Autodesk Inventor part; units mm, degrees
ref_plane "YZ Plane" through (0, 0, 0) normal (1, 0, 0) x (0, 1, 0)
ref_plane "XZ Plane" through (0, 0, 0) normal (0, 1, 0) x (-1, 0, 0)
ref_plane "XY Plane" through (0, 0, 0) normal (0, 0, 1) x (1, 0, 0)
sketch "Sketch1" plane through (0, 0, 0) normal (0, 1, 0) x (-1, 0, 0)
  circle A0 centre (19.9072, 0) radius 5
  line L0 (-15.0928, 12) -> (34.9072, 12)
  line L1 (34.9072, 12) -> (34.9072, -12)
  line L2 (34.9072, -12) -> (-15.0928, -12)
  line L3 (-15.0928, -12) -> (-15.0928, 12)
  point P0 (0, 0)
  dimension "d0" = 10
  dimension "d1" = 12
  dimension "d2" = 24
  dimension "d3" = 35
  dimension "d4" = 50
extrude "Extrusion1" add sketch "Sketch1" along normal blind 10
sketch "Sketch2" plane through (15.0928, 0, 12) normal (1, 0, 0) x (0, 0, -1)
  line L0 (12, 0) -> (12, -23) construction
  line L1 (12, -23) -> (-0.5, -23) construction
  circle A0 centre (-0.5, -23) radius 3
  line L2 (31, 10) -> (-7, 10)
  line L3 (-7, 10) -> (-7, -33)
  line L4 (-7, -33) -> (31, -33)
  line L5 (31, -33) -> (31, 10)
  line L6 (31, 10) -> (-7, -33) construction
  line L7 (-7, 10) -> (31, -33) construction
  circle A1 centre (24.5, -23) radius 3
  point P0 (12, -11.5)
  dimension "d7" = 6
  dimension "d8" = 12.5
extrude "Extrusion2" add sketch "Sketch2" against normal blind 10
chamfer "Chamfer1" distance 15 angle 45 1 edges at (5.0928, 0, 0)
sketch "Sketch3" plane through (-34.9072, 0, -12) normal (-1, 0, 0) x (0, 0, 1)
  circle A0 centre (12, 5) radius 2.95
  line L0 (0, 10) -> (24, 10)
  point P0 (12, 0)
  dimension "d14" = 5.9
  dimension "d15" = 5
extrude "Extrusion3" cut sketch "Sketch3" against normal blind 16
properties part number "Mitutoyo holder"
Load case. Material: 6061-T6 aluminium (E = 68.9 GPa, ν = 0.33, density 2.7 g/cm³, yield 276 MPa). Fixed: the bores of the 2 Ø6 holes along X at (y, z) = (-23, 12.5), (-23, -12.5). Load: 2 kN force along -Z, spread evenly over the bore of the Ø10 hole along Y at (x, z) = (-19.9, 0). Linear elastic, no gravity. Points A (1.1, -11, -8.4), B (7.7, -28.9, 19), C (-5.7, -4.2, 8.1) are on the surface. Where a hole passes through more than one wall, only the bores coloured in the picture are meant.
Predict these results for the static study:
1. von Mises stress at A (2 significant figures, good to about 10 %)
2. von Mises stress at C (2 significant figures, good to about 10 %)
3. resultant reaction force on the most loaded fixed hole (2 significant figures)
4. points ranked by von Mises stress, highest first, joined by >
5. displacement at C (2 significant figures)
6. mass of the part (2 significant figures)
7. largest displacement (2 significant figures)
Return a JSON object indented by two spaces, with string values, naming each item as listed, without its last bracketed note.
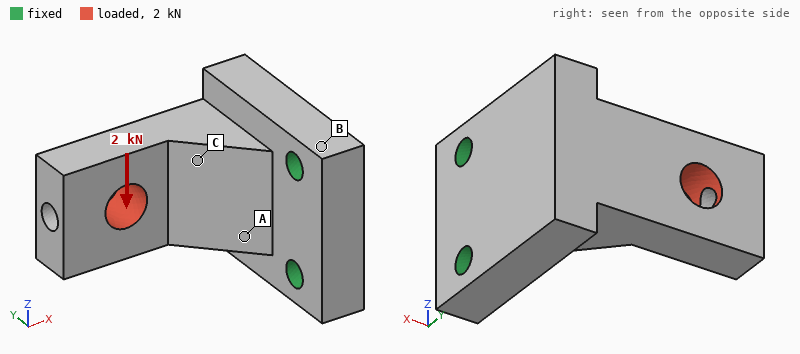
{
  "von Mises stress at A": "45 MPa",
  "von Mises stress at C": "31 MPa",
  "resultant reaction force on the most loaded fixed hole": "3.1 kN",
  "points ranked by von Mises stress, highest first, joined by >": "A > C > B",
  "displacement at C": "0.032 mm",
  "mass of the part": "73 g",
  "largest displacement": "0.11 mm"
}
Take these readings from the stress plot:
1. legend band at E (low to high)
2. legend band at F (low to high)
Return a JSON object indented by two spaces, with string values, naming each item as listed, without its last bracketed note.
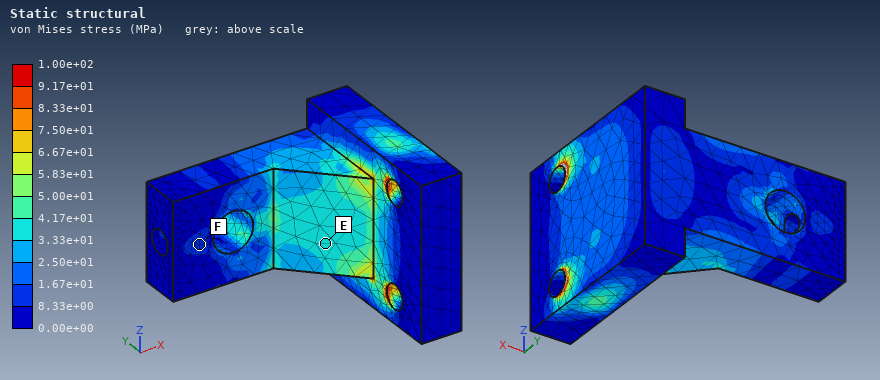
{
  "legend band at E": "3.33e+01 to 4.17e+01 MPa",
  "legend band at F": "8.33e+00 to 1.67e+01 MPa"
}
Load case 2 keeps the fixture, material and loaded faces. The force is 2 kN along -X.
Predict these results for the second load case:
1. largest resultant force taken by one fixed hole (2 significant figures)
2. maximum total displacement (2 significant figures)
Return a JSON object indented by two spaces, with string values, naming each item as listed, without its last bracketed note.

{
  "largest resultant force taken by one fixed hole": "1.0 kN",
  "maximum total displacement": "0.15 mm"
}
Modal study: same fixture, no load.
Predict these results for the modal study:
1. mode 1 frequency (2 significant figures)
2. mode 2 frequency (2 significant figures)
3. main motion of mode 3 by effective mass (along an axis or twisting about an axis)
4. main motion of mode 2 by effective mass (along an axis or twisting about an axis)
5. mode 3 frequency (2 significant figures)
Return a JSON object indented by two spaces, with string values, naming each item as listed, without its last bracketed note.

{
  "mode 1 frequency": "3200 Hz",
  "mode 2 frequency": "5700 Hz",
  "main motion of mode 3 by effective mass": "along X",
  "main motion of mode 2 by effective mass": "along Z",
  "mode 3 frequency": "9200 Hz"
}
